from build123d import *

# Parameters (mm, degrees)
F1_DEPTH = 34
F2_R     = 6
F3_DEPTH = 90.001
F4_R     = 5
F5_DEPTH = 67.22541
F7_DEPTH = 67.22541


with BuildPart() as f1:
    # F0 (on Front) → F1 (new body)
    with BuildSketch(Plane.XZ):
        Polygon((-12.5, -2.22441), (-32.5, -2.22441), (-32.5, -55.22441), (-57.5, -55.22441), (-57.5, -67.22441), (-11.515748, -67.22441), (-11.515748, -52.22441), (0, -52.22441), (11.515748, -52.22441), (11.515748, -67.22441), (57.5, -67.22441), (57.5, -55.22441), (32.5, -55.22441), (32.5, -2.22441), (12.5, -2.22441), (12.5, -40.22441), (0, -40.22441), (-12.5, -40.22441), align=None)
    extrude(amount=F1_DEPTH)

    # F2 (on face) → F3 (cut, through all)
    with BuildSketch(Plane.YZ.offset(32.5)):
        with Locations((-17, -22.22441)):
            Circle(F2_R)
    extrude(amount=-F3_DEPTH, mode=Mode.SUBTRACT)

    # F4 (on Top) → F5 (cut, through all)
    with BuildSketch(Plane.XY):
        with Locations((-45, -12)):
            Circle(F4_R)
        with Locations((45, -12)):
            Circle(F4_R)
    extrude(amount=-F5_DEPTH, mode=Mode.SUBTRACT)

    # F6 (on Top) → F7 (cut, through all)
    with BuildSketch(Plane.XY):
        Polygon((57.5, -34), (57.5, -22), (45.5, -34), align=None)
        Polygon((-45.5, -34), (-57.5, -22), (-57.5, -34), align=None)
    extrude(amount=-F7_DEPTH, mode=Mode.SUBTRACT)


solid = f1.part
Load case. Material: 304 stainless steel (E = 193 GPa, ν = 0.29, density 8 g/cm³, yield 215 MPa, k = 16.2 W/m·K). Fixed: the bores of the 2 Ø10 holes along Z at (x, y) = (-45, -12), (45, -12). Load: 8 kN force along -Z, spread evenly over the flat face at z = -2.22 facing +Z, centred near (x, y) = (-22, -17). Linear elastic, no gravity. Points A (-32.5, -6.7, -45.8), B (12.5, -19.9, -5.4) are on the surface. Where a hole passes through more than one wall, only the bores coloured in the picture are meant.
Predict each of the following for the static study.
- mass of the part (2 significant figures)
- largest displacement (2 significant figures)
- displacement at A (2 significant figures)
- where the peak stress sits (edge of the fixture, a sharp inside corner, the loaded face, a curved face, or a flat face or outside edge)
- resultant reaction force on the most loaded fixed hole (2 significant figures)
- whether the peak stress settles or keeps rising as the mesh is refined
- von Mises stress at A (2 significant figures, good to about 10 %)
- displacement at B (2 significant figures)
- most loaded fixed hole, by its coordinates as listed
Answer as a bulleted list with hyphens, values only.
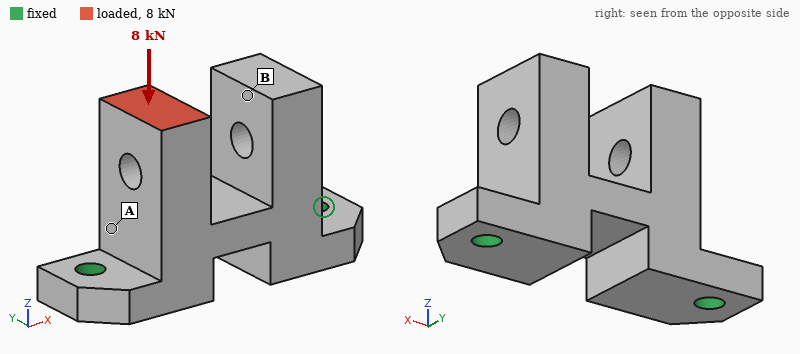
- 890 g
- 21 µm
- 7.5 µm
- edge of the fixture
- 7.2 kN
- keeps rising
- 21 MPa
- 11 µm
- (-45, -12)
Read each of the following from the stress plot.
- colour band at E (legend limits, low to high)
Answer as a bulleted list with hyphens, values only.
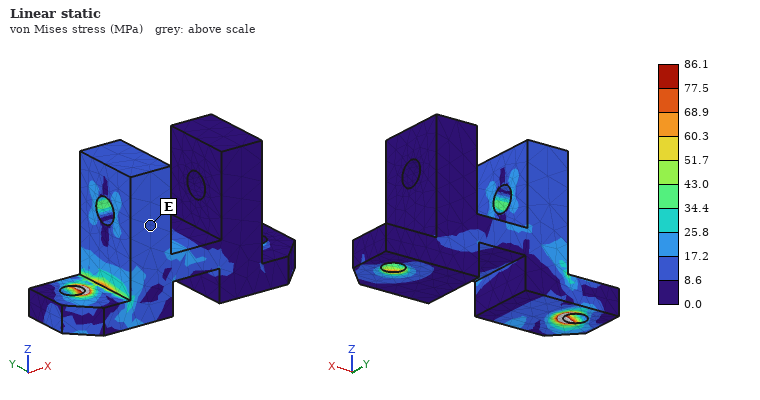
- 8.6 to 17.2 MPa
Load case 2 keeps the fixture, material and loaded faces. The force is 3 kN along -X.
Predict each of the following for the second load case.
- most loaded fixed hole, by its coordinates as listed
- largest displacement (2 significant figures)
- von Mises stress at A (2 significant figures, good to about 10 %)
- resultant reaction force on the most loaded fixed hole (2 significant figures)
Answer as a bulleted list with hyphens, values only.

- (45, -12)
- 47 µm
- 40 MPa
- 5.2 kN
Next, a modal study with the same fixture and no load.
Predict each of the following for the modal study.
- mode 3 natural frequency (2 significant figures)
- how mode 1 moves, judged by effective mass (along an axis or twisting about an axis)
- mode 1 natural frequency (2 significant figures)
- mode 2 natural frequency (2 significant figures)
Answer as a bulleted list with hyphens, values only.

- 4700 Hz
- along Y
- 2200 Hz
- 3900 Hz
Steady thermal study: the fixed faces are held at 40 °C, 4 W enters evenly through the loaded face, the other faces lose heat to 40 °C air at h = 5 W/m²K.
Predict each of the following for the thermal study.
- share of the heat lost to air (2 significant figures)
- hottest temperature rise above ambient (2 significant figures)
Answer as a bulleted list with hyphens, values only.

- 19 %
- 26 K
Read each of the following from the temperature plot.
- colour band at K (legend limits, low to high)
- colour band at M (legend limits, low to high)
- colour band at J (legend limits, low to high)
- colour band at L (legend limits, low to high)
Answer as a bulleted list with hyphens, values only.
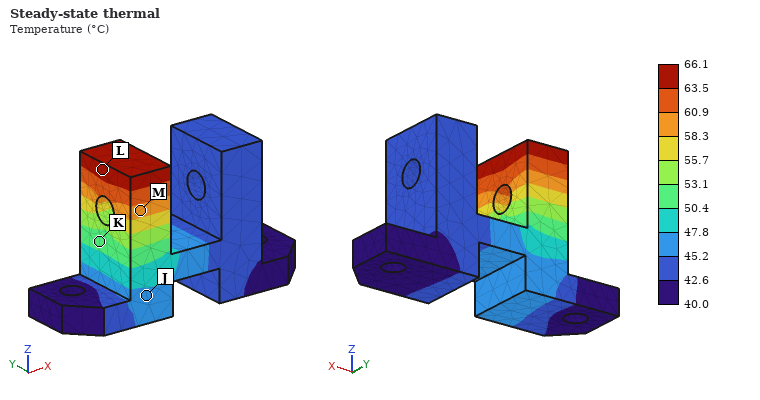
- 50.4 to 53.1 °C
- 58.3 to 60.9 °C
- 45.2 to 47.8 °C
- 63.5 to 66.1 °C
